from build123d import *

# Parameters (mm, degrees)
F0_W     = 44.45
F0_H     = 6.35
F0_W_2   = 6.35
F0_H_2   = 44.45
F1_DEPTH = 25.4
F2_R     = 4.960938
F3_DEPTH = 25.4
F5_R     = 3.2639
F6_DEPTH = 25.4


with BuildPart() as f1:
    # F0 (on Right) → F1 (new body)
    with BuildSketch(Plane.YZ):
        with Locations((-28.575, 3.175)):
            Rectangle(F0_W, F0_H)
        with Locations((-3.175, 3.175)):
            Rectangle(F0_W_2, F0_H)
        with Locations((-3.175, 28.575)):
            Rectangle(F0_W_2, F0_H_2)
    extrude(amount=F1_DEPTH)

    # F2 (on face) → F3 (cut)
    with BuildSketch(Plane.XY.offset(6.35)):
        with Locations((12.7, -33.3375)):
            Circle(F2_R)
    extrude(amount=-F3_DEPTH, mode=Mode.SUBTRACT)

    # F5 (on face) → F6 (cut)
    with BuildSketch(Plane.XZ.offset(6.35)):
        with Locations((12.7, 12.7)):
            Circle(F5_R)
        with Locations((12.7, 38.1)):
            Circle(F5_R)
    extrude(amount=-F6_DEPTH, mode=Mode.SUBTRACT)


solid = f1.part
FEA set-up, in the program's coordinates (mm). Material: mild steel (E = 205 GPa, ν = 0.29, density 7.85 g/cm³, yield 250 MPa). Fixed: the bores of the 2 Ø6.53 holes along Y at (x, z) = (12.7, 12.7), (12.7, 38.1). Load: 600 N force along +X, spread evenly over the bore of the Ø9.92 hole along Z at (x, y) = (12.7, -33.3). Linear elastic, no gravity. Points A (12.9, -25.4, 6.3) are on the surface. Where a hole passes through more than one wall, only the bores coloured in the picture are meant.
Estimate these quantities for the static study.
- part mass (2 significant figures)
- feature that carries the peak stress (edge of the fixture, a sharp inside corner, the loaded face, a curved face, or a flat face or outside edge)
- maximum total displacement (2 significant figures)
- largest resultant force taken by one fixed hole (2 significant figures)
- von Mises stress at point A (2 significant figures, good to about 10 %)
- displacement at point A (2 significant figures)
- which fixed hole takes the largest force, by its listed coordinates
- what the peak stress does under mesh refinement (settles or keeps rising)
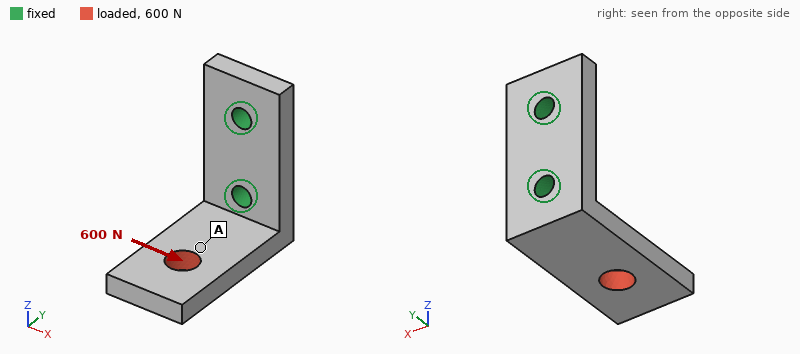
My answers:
110 g
edge of the fixture
45 µm
720 N
16 MPa
20 µm
(12.7, 12.7)
keeps rising
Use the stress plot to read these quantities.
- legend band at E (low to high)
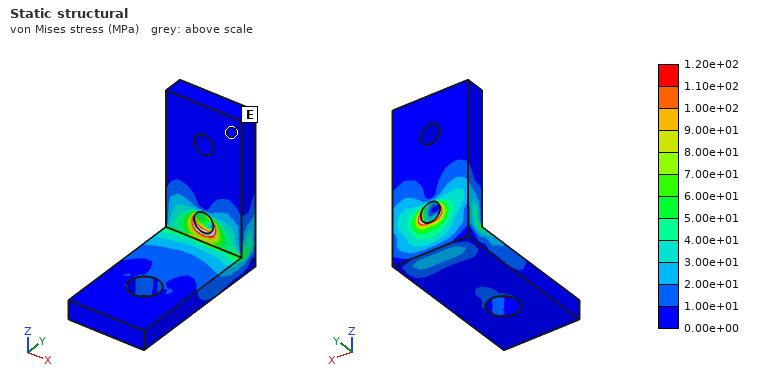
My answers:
0.00e+00 to 1.00e+01 MPa
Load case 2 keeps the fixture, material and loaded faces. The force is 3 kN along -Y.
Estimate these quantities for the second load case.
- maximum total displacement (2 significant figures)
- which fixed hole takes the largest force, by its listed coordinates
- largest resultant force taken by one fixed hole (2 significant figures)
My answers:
56 µm
(12.7, 12.7)
3.2 kN
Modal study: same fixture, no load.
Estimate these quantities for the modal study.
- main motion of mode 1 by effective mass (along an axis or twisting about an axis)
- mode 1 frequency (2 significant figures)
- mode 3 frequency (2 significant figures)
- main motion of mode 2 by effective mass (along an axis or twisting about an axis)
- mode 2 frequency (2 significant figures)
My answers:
along Z
1900 Hz
7600 Hz
along X
3400 Hz
